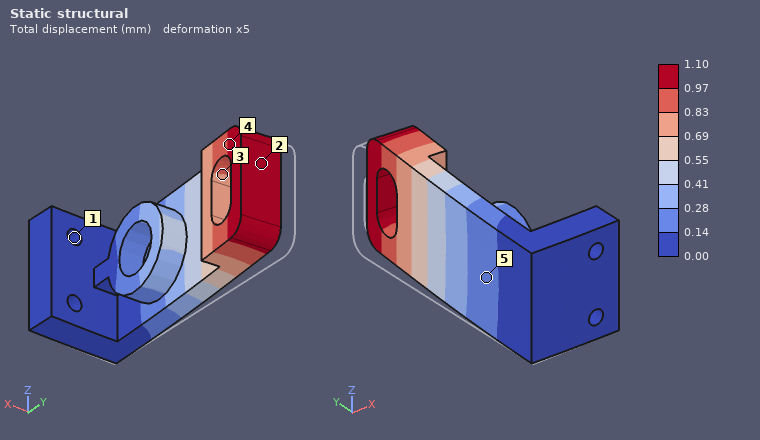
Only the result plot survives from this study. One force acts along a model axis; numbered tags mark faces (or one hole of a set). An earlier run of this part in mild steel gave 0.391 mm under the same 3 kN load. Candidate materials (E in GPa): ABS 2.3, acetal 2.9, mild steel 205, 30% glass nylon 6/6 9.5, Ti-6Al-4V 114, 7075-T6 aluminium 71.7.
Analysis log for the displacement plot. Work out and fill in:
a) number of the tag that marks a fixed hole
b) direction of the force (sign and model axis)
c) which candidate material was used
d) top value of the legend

1
+X
7075-T6 aluminium
1.10 mm
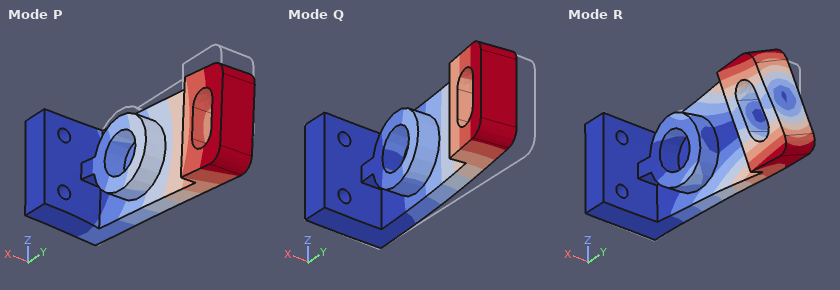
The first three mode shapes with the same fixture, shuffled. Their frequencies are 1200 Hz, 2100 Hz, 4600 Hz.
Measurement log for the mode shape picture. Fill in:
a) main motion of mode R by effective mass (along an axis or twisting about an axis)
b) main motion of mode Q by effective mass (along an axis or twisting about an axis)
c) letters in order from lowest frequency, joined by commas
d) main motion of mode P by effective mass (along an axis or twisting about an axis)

twisting about Y
along X
Q, P, R
along Z
